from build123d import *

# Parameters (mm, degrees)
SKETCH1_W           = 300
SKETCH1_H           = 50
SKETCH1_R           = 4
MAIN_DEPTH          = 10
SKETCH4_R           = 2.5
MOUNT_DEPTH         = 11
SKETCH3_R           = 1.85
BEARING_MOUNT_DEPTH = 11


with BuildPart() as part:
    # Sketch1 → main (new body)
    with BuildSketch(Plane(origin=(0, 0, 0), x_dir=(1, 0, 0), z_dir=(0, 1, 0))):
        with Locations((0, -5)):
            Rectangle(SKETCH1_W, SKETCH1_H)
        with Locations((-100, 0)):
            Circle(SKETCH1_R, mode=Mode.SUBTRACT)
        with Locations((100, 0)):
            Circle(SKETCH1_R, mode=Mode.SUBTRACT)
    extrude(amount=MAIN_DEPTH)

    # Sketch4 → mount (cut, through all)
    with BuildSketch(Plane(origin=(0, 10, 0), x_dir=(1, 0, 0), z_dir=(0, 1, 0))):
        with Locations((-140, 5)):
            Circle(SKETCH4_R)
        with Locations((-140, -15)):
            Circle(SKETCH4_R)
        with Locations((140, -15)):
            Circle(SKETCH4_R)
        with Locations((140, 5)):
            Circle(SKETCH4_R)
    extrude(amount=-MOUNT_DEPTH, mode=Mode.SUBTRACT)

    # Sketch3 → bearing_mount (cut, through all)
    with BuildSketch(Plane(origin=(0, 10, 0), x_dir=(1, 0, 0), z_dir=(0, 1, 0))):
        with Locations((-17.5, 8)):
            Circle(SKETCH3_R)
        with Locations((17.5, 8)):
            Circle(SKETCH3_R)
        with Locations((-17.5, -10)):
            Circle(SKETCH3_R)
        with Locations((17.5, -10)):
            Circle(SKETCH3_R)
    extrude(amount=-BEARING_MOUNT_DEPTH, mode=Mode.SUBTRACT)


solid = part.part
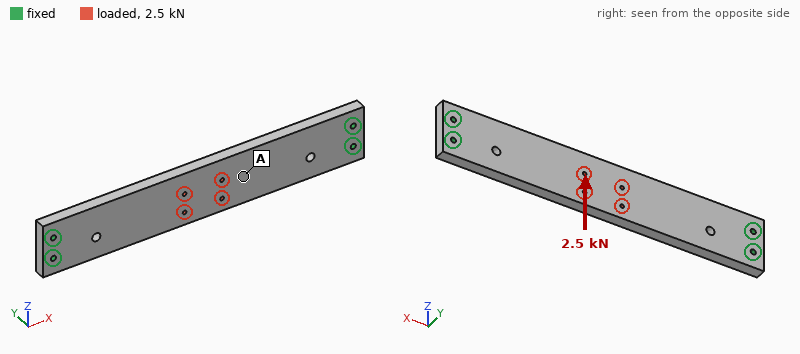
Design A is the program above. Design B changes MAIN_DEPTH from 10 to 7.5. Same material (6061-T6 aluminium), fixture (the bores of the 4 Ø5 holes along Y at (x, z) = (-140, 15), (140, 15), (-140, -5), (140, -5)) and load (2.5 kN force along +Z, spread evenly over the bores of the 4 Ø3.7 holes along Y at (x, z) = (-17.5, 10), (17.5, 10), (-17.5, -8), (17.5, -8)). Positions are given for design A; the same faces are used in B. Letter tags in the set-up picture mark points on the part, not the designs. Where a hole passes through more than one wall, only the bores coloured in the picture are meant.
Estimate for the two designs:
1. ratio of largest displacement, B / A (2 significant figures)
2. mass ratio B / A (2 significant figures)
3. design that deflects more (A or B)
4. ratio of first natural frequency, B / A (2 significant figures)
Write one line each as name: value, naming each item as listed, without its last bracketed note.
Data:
ratio of largest displacement, B / A: 1.3
mass ratio B / A: 0.75
design that deflects more: B
ratio of first natural frequency, B / A: 0.76
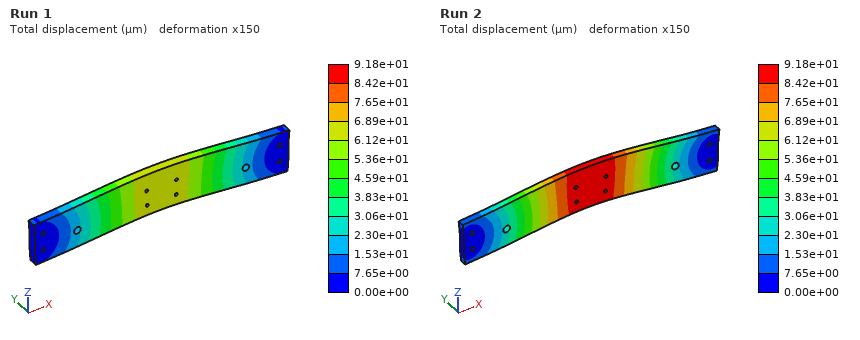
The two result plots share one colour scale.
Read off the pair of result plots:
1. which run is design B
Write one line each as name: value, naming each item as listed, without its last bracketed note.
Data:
which run is design B: Run 2
